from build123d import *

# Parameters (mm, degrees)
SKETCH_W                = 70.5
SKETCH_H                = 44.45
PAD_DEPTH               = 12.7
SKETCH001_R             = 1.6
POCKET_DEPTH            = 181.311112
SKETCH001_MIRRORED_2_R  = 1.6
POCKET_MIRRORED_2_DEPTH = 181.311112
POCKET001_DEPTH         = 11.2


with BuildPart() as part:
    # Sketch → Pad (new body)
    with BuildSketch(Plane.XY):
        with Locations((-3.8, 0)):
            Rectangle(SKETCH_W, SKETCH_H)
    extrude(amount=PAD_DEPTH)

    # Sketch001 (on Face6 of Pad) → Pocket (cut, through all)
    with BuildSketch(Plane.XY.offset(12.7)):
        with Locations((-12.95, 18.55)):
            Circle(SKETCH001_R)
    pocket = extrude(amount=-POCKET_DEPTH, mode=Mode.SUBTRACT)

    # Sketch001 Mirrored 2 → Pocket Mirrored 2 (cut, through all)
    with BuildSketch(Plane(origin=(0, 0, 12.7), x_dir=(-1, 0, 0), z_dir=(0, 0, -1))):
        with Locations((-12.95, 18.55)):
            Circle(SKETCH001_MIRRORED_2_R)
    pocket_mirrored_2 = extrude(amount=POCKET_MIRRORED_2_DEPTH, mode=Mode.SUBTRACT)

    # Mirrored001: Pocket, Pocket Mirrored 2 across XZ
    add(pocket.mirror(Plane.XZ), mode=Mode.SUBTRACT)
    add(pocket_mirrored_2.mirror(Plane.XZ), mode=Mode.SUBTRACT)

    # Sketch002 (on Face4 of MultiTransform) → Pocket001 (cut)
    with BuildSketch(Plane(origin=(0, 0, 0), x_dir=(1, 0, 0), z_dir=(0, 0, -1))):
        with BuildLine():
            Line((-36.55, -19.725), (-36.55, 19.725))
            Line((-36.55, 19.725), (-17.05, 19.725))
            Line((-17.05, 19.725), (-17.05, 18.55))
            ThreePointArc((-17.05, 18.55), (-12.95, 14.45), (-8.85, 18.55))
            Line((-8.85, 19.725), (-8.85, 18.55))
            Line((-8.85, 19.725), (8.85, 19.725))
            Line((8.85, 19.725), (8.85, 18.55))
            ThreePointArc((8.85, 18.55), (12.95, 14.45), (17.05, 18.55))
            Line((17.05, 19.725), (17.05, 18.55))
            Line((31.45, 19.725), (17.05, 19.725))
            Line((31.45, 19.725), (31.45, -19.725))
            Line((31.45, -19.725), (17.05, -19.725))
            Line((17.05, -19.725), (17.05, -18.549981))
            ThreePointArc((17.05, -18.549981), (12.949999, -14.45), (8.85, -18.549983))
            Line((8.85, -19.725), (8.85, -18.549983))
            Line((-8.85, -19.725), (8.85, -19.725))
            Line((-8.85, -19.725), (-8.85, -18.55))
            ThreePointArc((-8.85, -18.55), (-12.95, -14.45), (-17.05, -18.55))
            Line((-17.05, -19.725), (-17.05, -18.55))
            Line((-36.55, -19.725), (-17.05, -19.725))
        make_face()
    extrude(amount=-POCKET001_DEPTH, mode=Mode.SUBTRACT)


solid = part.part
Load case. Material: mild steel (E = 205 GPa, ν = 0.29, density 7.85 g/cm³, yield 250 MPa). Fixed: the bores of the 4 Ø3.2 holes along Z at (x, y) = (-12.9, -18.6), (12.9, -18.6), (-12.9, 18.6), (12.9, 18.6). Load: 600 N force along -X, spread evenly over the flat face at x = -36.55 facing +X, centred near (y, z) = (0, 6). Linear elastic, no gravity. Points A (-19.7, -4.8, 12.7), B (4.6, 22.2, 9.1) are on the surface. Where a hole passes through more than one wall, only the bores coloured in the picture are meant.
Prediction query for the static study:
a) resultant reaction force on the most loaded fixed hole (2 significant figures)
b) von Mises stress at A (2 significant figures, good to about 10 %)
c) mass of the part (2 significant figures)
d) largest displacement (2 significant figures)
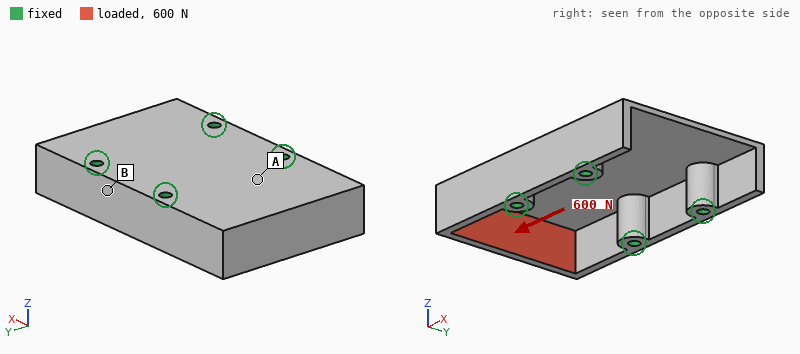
270 N
11 MPa
86 g
28 µm
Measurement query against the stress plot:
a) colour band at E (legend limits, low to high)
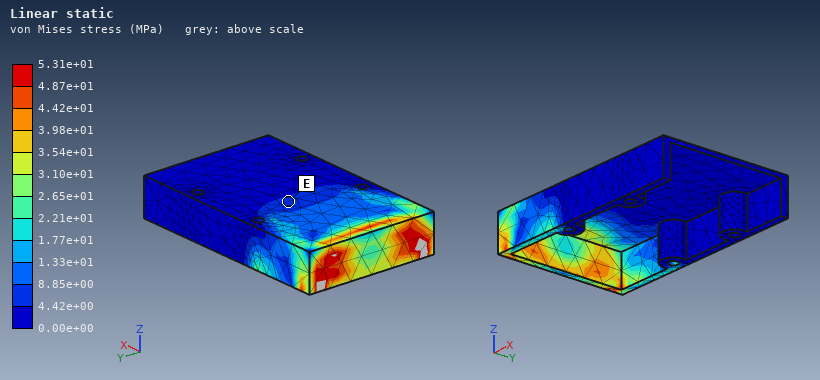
4.42e+00 to 8.85e+00 MPa
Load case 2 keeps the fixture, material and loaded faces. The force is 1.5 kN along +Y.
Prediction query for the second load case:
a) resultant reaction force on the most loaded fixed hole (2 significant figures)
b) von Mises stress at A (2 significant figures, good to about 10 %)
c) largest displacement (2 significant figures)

1.1 kN
35 MPa
28 µm
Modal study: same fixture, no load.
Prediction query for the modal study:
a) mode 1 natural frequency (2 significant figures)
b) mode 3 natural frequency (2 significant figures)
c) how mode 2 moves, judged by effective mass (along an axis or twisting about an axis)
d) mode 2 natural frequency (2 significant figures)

5600 Hz
7400 Hz
along Z
7000 Hz
